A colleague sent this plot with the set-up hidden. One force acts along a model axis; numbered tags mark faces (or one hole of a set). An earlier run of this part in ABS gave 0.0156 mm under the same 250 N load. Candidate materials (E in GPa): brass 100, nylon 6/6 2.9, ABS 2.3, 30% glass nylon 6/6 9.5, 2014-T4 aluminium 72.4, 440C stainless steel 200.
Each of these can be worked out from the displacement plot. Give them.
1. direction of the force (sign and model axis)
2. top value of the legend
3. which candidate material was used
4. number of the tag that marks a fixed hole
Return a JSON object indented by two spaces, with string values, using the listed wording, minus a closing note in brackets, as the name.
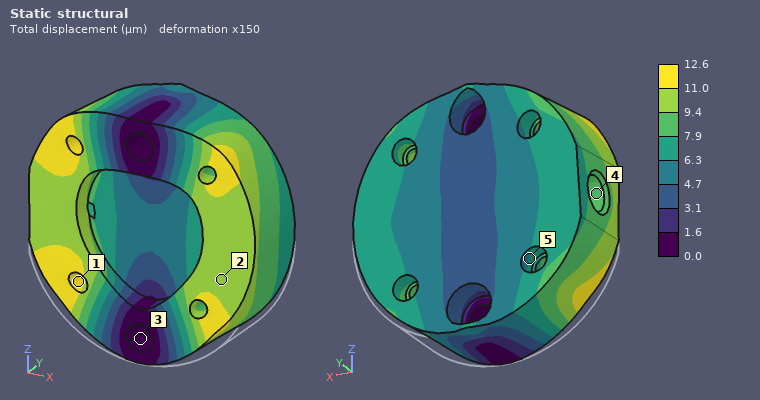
{
  "direction of the force": "+Z",
  "top value of the legend": "12.6 µm",
  "which candidate material was used": "nylon 6/6",
  "number of the tag that marks a fixed hole": "3"
}
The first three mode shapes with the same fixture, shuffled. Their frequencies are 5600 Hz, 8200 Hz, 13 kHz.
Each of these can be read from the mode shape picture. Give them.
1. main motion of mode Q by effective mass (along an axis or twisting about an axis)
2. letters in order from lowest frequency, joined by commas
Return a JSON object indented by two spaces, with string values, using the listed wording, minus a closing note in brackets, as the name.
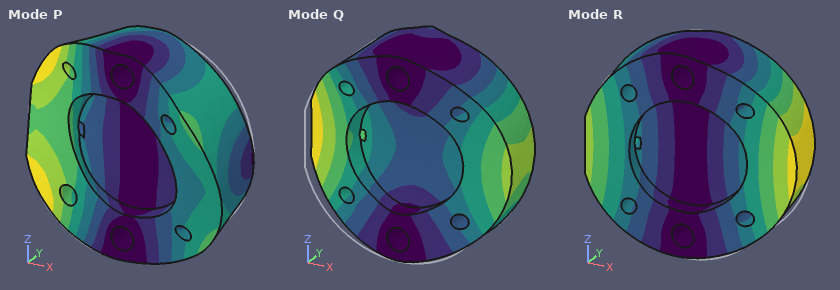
{
  "main motion of mode Q by effective mass": "along Y",
  "letters in order from lowest frequency, joined by commas": "R, Q, P"
}
